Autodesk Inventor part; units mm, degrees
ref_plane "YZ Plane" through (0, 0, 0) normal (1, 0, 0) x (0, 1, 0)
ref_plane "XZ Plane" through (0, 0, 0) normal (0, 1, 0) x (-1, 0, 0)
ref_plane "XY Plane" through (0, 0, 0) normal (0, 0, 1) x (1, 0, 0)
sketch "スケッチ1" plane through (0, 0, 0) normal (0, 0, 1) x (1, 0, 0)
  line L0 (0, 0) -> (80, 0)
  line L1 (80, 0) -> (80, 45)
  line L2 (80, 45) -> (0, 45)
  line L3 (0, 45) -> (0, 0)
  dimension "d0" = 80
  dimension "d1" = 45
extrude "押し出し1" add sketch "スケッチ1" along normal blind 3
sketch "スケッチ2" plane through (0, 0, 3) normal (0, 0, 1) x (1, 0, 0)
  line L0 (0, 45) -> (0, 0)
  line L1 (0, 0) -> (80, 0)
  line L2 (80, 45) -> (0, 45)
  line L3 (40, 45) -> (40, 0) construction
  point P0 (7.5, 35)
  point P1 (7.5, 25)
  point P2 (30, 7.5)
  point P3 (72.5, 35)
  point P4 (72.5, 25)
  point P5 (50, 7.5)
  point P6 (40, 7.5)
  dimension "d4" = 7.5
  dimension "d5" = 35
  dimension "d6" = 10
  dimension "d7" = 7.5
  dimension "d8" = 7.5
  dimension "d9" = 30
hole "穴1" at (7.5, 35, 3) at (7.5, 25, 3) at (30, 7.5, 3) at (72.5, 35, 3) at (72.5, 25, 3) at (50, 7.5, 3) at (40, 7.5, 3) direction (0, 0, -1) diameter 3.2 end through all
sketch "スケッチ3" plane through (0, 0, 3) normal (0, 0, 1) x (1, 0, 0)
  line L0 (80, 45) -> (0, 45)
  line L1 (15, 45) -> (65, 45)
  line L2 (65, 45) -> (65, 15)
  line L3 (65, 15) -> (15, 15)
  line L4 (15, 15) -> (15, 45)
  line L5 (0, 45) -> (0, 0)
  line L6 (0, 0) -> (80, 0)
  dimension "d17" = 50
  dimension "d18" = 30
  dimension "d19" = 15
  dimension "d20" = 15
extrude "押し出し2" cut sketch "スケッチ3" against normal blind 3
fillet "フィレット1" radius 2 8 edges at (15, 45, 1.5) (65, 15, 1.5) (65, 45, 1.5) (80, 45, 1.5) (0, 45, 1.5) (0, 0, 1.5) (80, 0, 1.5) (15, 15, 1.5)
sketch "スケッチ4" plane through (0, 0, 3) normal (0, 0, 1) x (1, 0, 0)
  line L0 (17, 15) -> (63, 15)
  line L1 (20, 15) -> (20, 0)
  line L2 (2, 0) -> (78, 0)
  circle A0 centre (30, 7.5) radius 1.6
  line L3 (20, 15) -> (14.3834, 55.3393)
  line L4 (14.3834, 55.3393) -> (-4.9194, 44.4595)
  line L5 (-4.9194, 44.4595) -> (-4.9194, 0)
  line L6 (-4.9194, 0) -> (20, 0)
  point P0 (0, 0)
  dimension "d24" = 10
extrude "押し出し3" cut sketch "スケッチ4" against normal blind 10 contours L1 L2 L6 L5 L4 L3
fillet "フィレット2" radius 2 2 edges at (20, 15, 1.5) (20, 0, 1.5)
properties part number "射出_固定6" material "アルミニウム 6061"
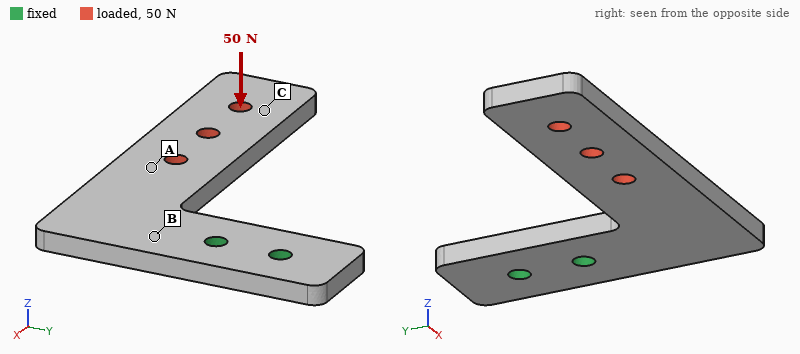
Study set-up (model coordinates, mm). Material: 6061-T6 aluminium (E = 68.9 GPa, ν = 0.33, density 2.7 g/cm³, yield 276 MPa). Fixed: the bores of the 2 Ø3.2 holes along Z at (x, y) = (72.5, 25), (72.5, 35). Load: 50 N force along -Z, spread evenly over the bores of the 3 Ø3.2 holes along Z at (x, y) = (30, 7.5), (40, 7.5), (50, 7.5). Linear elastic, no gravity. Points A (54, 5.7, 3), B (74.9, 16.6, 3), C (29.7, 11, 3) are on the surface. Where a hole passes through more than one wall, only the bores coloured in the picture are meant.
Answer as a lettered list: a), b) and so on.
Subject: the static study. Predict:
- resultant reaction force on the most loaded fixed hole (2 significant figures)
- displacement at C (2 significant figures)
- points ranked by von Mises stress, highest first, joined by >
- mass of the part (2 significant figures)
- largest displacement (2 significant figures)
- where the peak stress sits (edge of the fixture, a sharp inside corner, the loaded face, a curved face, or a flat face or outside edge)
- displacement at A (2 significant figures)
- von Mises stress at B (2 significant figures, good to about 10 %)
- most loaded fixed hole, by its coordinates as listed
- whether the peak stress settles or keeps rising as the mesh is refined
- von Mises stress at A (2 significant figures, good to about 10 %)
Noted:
a) 75 N
b) 0.59 mm
c) B > A > C
d) 11 g
e) 0.80 mm
f) edge of the fixture
g) 0.23 mm
h) 54 MPa
i) (72.5, 25)
j) keeps rising
k) 31 MPa
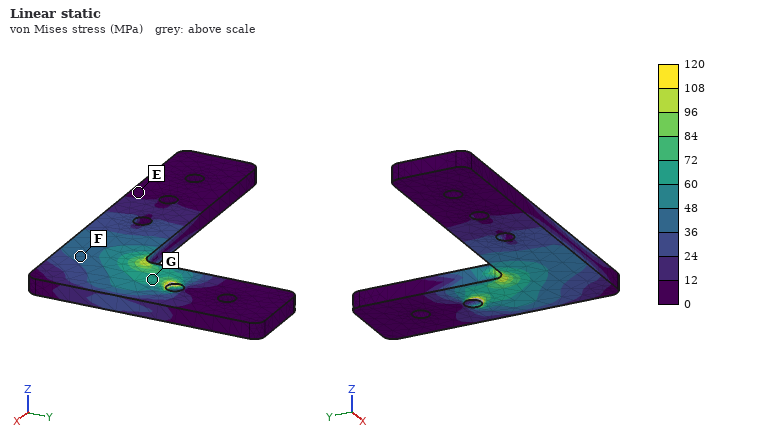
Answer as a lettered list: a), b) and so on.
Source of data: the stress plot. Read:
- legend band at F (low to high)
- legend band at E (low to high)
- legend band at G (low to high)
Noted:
a) 36 to 48 MPa
b) 0 to 12 MPa
c) 60 to 72 MPa
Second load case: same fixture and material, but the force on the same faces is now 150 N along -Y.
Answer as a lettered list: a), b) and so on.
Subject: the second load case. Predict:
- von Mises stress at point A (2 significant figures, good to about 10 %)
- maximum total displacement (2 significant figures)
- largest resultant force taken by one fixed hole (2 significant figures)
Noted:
a) 8.8 MPa
b) 0.15 mm
c) 340 N
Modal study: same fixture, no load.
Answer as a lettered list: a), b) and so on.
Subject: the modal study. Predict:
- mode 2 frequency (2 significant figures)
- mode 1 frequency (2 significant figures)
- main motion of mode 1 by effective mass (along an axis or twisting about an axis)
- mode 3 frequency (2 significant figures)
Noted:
a) 2700 Hz
b) 710 Hz
c) along Z
d) 2700 Hz
